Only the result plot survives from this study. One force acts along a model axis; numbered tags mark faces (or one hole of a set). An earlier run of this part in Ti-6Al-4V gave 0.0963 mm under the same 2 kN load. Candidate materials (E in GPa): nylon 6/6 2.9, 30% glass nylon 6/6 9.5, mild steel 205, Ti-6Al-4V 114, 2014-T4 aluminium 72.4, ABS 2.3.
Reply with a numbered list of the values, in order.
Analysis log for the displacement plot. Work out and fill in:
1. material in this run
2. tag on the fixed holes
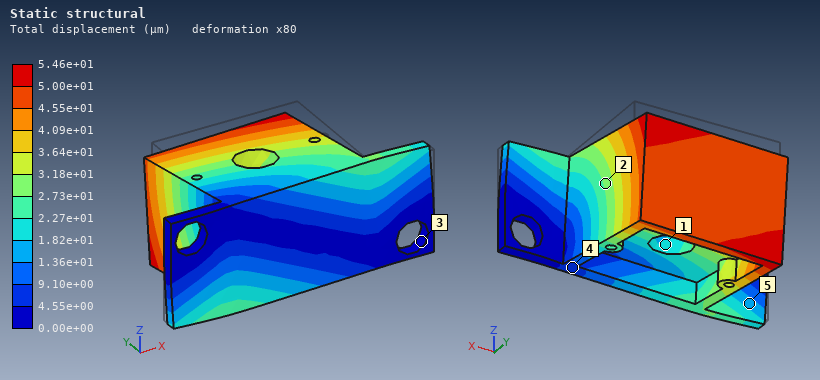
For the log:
1. mild steel
2. 3
